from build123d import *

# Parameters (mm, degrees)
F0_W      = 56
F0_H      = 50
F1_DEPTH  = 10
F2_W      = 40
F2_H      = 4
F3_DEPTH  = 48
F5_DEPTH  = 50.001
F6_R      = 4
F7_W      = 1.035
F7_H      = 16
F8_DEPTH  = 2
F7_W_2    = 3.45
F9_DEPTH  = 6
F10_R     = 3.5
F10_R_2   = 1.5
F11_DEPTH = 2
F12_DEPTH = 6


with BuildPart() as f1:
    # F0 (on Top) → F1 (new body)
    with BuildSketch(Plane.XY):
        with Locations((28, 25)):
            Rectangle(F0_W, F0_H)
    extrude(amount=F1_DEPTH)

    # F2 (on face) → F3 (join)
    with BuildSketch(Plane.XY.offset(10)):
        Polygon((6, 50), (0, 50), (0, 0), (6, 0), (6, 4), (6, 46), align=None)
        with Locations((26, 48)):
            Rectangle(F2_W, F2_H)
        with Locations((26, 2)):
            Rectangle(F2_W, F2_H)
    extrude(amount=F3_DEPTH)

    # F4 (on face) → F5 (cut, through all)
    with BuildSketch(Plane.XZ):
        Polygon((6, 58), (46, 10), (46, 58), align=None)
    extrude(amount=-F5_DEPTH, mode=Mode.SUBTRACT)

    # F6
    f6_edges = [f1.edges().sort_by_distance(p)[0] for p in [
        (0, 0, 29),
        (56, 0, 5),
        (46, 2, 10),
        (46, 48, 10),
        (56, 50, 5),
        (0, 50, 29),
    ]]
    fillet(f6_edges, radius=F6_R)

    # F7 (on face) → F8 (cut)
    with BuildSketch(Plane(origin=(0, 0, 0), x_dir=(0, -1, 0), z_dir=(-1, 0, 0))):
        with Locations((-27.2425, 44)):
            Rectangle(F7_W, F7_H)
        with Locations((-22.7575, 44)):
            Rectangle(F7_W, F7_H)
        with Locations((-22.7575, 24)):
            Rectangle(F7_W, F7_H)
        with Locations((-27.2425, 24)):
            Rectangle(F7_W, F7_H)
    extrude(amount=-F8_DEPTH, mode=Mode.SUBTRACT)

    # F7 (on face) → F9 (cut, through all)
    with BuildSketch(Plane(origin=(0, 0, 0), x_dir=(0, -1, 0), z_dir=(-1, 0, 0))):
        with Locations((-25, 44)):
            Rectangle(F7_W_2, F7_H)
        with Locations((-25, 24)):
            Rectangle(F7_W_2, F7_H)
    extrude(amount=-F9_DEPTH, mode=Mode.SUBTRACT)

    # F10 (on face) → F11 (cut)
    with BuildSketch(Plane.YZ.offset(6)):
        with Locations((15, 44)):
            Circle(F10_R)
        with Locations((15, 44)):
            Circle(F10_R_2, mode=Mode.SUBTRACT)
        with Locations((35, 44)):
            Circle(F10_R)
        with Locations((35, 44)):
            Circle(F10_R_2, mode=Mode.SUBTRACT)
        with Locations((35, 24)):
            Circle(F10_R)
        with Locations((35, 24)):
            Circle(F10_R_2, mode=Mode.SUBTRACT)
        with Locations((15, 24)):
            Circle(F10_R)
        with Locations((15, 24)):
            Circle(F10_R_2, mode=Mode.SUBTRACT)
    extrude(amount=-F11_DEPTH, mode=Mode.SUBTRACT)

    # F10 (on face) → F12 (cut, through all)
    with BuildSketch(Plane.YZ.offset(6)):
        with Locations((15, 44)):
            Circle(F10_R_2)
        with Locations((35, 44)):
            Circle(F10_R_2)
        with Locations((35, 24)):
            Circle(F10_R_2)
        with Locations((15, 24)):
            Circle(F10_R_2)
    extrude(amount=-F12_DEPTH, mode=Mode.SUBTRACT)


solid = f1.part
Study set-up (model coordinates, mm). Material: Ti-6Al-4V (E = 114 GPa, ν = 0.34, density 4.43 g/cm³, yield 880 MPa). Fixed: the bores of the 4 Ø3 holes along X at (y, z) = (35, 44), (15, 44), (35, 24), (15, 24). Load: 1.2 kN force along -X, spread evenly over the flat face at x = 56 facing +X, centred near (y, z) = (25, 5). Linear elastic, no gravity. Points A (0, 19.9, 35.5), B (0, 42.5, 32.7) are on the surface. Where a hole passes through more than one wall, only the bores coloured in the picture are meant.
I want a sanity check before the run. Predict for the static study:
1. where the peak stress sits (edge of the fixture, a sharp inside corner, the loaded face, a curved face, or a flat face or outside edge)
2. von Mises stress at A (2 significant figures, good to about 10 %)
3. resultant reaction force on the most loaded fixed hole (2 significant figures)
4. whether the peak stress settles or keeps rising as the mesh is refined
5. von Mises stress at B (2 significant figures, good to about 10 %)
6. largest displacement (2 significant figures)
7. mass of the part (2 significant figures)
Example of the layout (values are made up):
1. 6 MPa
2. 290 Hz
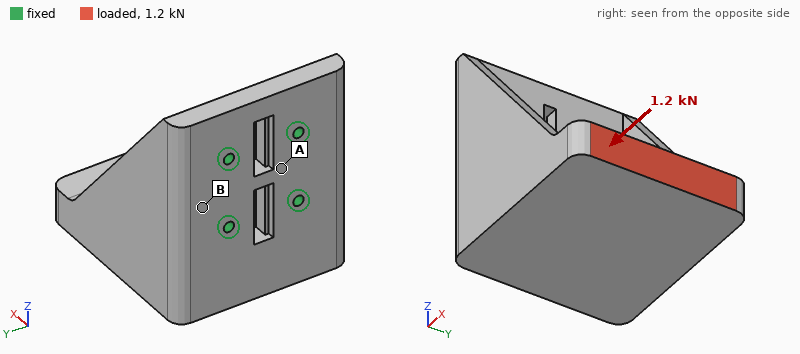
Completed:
1. edge of the fixture
2. 5.0 MPa
3. 1.1 kN
4. keeps rising
5. 15 MPa
6. 45 µm
7. 210 g
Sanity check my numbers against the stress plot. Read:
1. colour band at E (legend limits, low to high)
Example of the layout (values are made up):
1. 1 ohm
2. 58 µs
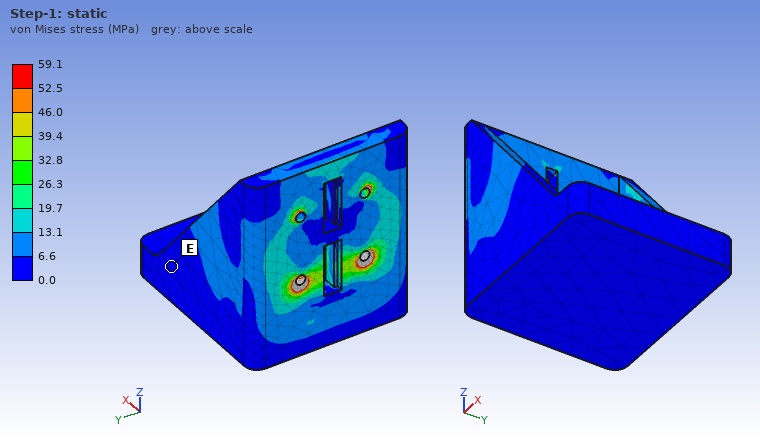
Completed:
1. 0.0 to 6.6 MPa
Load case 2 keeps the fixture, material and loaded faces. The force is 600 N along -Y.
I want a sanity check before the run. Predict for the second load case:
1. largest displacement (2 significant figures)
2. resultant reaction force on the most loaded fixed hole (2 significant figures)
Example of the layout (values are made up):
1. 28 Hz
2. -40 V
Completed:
1. 69 µm
2. 1.1 kN
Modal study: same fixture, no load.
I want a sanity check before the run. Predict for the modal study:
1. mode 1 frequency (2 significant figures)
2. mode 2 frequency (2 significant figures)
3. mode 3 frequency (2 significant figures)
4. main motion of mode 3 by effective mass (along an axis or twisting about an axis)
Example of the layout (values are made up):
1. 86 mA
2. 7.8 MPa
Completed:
1. 2100 Hz
2. 2100 Hz
3. 5800 Hz
4. along X
